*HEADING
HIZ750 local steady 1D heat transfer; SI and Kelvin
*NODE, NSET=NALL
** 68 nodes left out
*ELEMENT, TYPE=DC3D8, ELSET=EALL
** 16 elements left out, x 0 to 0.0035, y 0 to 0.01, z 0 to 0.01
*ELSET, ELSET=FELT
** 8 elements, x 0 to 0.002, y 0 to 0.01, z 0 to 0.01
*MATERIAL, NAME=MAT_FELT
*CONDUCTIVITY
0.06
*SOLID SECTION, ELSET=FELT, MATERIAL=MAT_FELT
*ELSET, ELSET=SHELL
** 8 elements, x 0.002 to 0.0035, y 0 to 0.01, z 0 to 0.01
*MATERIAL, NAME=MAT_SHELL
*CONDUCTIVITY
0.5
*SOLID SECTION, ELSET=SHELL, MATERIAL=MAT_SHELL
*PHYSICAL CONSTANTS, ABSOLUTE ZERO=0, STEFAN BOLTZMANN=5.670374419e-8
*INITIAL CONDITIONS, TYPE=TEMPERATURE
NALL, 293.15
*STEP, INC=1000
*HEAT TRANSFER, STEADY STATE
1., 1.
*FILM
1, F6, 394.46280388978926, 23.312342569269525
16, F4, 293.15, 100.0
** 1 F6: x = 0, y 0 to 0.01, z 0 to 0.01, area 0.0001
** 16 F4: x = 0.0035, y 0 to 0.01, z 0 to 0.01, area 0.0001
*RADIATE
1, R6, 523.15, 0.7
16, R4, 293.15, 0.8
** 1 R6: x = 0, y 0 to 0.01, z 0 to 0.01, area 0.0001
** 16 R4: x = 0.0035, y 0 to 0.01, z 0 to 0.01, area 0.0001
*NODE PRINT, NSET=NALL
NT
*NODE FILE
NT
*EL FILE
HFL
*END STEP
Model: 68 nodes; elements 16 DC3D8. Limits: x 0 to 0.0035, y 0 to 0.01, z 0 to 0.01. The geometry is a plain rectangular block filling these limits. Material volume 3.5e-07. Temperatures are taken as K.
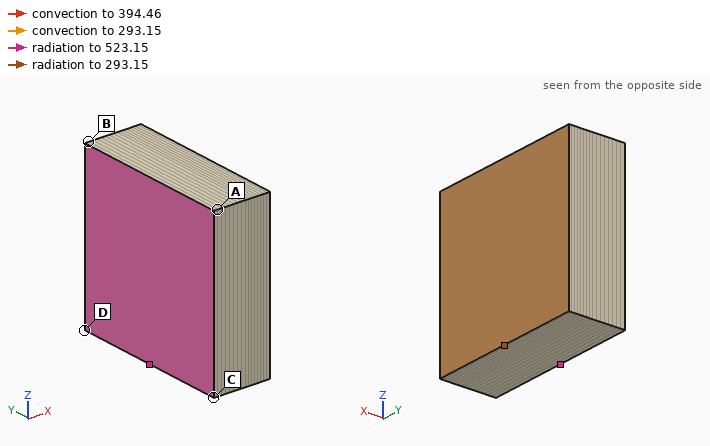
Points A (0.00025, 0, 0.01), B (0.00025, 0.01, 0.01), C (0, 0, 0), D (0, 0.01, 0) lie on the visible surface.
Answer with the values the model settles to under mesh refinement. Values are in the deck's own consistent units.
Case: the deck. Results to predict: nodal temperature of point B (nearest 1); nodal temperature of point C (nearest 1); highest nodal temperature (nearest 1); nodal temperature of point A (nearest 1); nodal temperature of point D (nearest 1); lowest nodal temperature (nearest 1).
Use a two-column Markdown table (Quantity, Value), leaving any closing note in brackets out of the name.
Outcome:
| Quantity | Value |
|---|---|
| nodal temperature of point B | 382 K |
| nodal temperature of point C | 391 K |
| highest nodal temperature | 391 K |
| nodal temperature of point A | 382 K |
| nodal temperature of point D | 391 K |
| lowest nodal temperature | 313 K |
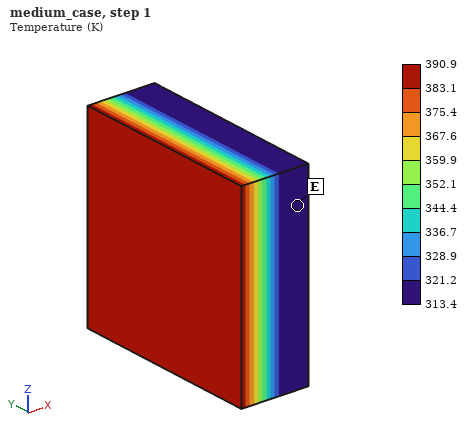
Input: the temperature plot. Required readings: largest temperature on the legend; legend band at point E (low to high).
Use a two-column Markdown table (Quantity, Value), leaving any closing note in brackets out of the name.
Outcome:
| Quantity | Value |
|---|---|
| largest temperature on the legend | 390.9 K |
| legend band at point E | 313.4 to 321.2 K |
